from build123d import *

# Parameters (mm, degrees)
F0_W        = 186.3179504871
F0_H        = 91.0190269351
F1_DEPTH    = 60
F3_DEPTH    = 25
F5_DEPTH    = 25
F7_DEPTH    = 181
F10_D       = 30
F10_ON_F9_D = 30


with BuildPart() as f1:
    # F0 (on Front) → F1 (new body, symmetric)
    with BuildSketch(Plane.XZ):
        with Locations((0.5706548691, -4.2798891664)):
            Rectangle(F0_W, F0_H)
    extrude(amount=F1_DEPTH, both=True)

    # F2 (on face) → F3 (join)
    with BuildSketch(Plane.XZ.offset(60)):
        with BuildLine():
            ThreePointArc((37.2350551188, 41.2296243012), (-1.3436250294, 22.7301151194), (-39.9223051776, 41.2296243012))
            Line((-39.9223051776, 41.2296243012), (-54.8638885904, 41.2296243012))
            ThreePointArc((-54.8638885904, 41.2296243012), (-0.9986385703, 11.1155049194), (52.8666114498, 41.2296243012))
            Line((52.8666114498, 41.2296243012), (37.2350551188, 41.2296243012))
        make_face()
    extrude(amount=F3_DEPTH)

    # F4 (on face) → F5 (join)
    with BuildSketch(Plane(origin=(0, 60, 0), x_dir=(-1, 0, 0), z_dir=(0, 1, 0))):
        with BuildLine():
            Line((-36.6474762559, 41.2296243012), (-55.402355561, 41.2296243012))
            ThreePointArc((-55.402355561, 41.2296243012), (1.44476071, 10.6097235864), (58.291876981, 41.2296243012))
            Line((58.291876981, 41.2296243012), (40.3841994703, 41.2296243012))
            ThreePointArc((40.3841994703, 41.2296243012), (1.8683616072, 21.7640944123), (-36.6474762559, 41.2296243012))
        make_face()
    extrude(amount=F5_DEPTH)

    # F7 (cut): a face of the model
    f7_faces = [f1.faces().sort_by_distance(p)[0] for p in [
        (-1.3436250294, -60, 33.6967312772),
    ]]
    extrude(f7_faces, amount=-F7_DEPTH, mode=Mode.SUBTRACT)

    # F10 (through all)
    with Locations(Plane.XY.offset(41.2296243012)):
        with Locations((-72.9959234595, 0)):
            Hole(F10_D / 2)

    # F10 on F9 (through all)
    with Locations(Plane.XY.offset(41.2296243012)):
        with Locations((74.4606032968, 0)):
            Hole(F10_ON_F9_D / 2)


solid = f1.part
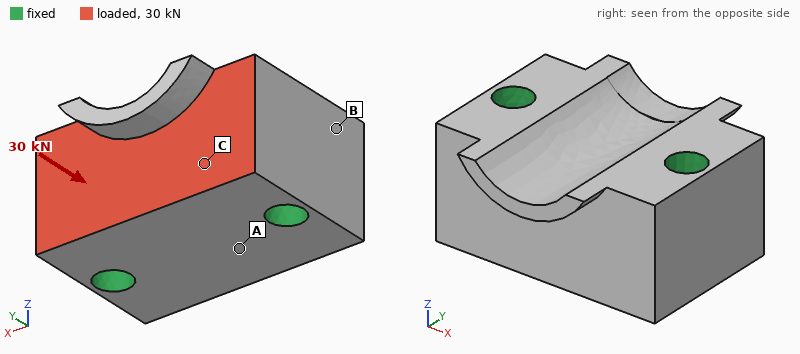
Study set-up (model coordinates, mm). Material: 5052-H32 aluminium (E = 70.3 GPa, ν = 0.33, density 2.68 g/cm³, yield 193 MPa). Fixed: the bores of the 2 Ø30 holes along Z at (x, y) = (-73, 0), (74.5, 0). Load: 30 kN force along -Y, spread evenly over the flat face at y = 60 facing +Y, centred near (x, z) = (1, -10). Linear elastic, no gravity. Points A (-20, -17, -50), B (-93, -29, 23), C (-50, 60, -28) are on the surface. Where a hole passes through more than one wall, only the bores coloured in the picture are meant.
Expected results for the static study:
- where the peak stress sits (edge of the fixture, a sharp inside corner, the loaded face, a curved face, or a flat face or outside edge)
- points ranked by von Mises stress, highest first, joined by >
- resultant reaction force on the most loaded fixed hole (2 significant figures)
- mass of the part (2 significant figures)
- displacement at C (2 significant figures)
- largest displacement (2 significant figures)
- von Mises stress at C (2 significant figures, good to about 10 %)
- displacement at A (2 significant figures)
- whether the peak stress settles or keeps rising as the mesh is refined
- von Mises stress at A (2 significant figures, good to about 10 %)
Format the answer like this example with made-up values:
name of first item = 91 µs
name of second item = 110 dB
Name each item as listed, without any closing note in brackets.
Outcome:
where the peak stress sits = edge of the fixture
points ranked by von Mises stress, highest first, joined by > = C > A > B
resultant reaction force on the most loaded fixed hole = 15 kN
mass of the part = 5.0 kg
displacement at C = 2.4 µm
largest displacement = 3.8 µm
von Mises stress at C = 2.0 MPa
displacement at A = 1.9 µm
whether the peak stress settles or keeps rising as the mesh is refined = keeps rising
von Mises stress at A = 1.1 MPa
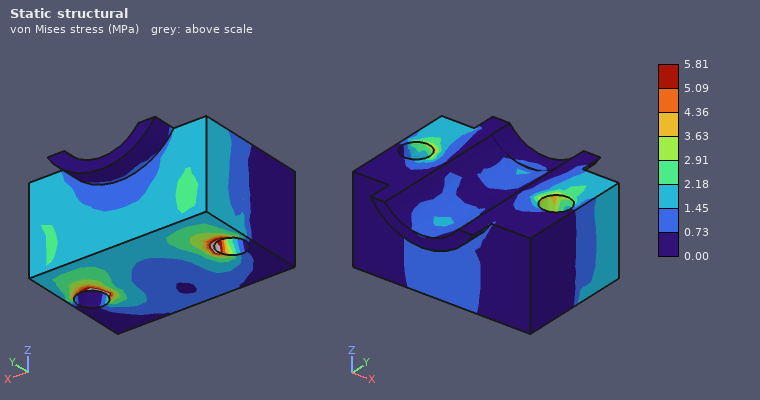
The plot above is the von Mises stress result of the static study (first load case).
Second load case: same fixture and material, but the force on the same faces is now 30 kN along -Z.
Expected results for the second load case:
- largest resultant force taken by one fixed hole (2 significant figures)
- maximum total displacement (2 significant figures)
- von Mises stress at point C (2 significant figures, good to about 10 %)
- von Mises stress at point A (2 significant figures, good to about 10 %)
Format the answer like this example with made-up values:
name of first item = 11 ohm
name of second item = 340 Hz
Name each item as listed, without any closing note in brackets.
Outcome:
largest resultant force taken by one fixed hole = 15 kN
maximum total displacement = 13 µm
von Mises stress at point C = 5.0 MPa
von Mises stress at point A = 2.3 MPa
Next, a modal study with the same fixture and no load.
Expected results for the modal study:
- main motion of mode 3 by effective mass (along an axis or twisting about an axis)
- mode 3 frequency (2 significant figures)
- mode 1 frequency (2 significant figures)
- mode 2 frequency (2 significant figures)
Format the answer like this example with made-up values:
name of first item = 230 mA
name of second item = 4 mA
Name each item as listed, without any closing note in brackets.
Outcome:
main motion of mode 3 by effective mass = along Y
mode 3 frequency = 9000 Hz
mode 1 frequency = 7700 Hz
mode 2 frequency = 7900 Hz
